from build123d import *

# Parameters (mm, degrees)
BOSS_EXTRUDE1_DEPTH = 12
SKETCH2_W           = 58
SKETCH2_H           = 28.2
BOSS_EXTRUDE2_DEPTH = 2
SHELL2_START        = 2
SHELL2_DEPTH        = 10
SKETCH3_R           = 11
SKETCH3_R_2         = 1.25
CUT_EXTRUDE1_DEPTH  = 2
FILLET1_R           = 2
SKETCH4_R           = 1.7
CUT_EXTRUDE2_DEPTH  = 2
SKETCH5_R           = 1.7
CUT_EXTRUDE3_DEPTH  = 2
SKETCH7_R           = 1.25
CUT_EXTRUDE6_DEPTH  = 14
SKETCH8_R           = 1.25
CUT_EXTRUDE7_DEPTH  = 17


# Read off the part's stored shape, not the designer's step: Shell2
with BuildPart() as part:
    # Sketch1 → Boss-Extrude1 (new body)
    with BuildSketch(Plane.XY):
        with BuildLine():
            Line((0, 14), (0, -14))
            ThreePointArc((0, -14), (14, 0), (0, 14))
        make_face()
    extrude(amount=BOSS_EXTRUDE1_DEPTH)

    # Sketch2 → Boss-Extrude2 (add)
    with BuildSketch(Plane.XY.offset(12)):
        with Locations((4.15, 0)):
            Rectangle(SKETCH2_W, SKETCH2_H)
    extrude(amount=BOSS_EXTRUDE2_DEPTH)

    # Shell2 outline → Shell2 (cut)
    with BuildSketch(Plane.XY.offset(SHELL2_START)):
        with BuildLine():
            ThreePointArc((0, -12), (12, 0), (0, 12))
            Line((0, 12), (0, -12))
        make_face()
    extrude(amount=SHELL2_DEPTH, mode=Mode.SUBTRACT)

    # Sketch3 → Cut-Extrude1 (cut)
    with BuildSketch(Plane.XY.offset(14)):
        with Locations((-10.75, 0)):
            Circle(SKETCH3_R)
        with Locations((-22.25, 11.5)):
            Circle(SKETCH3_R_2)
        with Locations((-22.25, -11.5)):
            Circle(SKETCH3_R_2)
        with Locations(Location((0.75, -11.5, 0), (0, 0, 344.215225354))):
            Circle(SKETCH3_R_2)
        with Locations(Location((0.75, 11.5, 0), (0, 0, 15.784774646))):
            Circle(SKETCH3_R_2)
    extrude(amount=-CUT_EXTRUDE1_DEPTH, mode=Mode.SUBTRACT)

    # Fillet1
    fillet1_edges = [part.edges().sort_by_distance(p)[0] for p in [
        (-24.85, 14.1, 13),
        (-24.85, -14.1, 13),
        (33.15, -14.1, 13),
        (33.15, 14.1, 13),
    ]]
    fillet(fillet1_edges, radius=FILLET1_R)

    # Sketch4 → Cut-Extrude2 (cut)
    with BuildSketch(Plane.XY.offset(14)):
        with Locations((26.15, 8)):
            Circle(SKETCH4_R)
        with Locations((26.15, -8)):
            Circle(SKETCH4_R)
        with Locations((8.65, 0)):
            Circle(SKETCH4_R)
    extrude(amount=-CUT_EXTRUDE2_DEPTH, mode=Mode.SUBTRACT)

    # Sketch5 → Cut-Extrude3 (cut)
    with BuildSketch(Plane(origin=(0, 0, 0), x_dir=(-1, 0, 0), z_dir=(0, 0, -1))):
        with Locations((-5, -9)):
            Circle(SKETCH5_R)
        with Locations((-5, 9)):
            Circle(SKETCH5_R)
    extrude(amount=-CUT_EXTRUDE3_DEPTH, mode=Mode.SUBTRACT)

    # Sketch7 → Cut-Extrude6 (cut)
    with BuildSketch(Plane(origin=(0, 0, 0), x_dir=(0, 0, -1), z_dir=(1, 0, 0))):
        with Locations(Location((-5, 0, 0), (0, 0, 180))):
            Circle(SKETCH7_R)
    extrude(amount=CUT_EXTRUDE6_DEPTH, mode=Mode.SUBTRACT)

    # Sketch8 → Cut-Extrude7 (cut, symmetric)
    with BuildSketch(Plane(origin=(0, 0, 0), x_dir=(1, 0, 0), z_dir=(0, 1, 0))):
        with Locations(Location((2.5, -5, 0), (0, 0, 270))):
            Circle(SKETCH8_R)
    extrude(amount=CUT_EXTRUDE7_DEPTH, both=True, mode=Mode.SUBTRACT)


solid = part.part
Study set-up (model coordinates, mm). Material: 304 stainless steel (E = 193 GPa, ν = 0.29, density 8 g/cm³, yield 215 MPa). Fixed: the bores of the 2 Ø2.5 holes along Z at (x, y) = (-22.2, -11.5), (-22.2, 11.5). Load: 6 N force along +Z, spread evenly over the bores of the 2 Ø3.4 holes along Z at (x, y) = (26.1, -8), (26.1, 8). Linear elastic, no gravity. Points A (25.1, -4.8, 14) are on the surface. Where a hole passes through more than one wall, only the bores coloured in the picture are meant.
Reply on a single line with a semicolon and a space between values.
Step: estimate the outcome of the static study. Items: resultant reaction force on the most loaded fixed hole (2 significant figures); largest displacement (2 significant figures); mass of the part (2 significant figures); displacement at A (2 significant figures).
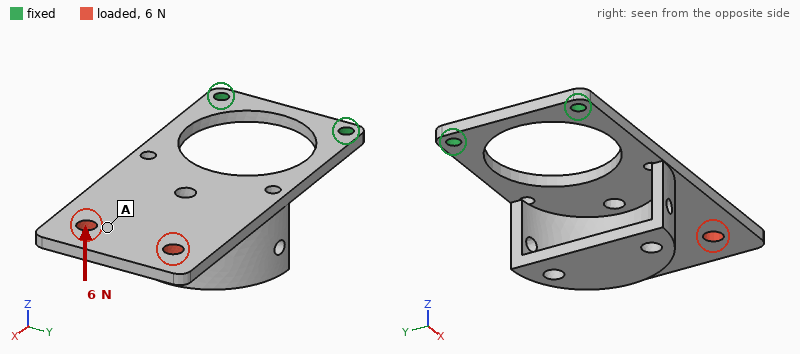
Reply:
3.0 N; 0.21 mm; 30 g; 0.17 mm
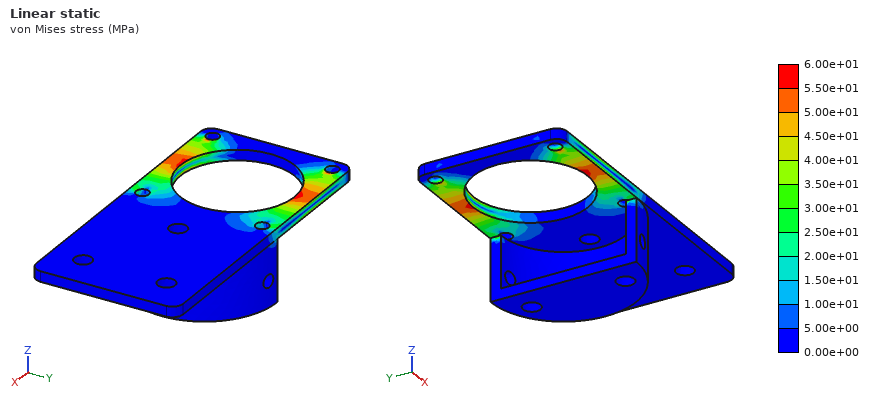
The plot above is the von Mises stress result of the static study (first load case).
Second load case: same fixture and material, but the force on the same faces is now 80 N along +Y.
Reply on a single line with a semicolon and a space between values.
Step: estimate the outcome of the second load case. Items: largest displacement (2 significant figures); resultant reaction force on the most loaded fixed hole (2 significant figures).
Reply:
18 µm; 140 N
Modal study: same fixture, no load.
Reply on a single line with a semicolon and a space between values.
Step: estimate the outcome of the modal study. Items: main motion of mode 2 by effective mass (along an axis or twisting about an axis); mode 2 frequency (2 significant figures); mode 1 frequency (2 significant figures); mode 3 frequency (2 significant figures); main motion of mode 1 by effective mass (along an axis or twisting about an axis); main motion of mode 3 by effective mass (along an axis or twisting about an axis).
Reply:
along Y; 1300 Hz; 270 Hz; 2300 Hz; along Z; along Z
